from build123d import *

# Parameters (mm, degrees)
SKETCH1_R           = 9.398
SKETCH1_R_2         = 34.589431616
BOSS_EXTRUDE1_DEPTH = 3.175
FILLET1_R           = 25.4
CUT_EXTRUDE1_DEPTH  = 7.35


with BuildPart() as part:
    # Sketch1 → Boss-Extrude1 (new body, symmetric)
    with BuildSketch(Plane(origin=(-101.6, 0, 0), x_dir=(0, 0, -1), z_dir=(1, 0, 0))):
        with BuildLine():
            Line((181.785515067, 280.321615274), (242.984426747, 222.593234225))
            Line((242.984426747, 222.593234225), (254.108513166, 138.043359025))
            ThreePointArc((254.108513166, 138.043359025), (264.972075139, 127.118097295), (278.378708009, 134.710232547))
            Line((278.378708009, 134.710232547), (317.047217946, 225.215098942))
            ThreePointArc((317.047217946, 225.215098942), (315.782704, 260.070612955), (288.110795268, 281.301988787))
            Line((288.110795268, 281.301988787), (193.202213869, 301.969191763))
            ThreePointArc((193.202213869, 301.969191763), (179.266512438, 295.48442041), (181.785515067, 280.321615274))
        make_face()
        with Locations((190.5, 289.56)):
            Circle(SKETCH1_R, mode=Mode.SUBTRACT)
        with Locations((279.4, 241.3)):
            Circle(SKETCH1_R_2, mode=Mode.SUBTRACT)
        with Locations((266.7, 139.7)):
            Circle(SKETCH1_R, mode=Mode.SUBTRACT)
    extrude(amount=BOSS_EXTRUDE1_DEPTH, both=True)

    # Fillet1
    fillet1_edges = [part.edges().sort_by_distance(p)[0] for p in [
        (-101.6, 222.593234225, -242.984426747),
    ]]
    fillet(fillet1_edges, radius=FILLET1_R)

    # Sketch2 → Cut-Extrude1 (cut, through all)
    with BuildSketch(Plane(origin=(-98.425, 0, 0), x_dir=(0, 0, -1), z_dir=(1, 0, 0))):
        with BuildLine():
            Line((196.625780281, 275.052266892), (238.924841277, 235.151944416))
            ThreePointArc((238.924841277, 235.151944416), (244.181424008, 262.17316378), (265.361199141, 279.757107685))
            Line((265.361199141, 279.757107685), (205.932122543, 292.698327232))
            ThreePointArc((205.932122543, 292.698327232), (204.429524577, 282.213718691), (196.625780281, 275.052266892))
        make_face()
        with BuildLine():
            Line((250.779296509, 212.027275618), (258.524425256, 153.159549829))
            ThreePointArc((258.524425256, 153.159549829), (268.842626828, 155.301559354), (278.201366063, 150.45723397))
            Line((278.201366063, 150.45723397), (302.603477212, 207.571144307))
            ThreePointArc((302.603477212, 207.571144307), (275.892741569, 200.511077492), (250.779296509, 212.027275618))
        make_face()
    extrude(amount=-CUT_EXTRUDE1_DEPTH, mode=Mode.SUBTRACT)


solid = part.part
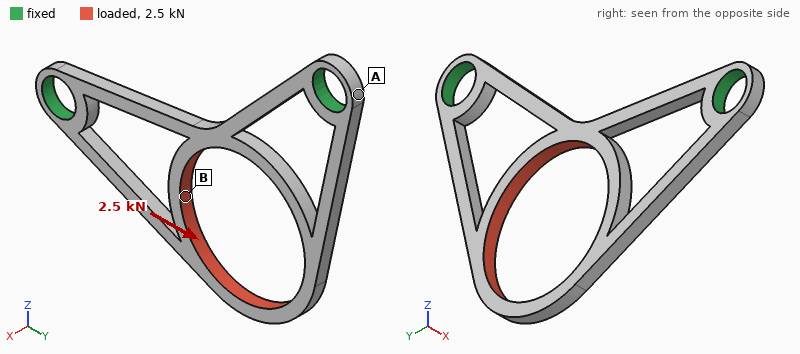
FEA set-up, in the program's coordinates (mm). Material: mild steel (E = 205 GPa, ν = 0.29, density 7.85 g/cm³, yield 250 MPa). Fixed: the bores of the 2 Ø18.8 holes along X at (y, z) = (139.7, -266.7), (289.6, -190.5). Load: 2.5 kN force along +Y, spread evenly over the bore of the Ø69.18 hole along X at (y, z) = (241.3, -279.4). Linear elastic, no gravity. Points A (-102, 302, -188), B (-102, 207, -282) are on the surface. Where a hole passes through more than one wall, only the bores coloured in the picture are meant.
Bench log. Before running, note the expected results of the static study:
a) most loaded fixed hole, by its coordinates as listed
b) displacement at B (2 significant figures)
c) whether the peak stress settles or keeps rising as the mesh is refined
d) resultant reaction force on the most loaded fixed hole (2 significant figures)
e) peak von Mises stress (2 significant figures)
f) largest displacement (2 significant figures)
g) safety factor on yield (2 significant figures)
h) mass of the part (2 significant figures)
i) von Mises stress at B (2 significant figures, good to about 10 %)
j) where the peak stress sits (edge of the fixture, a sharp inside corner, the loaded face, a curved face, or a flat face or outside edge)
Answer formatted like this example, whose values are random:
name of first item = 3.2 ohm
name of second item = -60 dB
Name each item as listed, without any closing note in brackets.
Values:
most loaded fixed hole, by its coordinates as listed = (139.7, -266.7)
displacement at B = 11 µm
whether the peak stress settles or keeps rising as the mesh is refined = settles
resultant reaction force on the most loaded fixed hole = 2.3 kN
peak von Mises stress = 90 MPa
largest displacement = 69 µm
safety factor on yield = 2.8
mass of the part = 200 g
von Mises stress at B = 39 MPa
where the peak stress sits = the loaded face
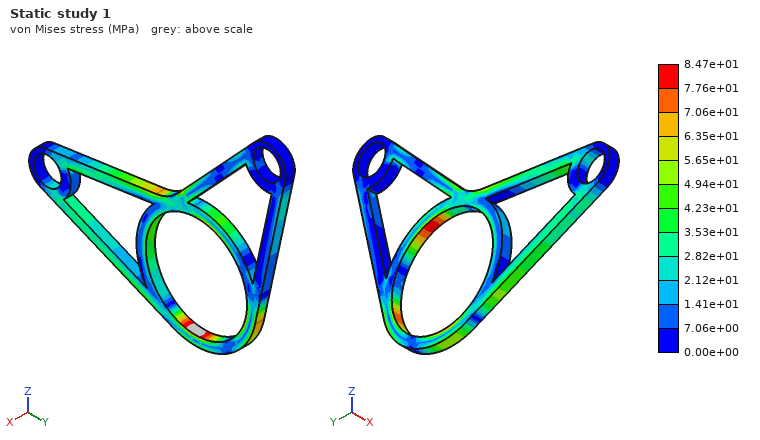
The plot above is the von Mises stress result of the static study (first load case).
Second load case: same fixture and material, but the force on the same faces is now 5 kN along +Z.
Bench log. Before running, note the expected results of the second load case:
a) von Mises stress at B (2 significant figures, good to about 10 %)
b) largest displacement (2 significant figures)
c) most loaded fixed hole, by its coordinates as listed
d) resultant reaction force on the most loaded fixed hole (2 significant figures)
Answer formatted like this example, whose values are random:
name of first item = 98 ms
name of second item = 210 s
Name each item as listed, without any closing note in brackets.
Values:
von Mises stress at B = 68 MPa
largest displacement = 0.11 mm
most loaded fixed hole, by its coordinates as listed = (289.6, -190.5)
resultant reaction force on the most loaded fixed hole = 5.1 kN
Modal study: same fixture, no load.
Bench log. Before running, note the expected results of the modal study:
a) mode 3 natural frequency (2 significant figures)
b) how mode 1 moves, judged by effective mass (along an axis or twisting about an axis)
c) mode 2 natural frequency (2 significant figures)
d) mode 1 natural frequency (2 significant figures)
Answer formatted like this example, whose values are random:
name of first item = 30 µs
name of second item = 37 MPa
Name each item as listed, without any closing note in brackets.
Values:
mode 3 natural frequency = 1300 Hz
how mode 1 moves, judged by effective mass = along X
mode 2 natural frequency = 1300 Hz
mode 1 natural frequency = 440 Hz
